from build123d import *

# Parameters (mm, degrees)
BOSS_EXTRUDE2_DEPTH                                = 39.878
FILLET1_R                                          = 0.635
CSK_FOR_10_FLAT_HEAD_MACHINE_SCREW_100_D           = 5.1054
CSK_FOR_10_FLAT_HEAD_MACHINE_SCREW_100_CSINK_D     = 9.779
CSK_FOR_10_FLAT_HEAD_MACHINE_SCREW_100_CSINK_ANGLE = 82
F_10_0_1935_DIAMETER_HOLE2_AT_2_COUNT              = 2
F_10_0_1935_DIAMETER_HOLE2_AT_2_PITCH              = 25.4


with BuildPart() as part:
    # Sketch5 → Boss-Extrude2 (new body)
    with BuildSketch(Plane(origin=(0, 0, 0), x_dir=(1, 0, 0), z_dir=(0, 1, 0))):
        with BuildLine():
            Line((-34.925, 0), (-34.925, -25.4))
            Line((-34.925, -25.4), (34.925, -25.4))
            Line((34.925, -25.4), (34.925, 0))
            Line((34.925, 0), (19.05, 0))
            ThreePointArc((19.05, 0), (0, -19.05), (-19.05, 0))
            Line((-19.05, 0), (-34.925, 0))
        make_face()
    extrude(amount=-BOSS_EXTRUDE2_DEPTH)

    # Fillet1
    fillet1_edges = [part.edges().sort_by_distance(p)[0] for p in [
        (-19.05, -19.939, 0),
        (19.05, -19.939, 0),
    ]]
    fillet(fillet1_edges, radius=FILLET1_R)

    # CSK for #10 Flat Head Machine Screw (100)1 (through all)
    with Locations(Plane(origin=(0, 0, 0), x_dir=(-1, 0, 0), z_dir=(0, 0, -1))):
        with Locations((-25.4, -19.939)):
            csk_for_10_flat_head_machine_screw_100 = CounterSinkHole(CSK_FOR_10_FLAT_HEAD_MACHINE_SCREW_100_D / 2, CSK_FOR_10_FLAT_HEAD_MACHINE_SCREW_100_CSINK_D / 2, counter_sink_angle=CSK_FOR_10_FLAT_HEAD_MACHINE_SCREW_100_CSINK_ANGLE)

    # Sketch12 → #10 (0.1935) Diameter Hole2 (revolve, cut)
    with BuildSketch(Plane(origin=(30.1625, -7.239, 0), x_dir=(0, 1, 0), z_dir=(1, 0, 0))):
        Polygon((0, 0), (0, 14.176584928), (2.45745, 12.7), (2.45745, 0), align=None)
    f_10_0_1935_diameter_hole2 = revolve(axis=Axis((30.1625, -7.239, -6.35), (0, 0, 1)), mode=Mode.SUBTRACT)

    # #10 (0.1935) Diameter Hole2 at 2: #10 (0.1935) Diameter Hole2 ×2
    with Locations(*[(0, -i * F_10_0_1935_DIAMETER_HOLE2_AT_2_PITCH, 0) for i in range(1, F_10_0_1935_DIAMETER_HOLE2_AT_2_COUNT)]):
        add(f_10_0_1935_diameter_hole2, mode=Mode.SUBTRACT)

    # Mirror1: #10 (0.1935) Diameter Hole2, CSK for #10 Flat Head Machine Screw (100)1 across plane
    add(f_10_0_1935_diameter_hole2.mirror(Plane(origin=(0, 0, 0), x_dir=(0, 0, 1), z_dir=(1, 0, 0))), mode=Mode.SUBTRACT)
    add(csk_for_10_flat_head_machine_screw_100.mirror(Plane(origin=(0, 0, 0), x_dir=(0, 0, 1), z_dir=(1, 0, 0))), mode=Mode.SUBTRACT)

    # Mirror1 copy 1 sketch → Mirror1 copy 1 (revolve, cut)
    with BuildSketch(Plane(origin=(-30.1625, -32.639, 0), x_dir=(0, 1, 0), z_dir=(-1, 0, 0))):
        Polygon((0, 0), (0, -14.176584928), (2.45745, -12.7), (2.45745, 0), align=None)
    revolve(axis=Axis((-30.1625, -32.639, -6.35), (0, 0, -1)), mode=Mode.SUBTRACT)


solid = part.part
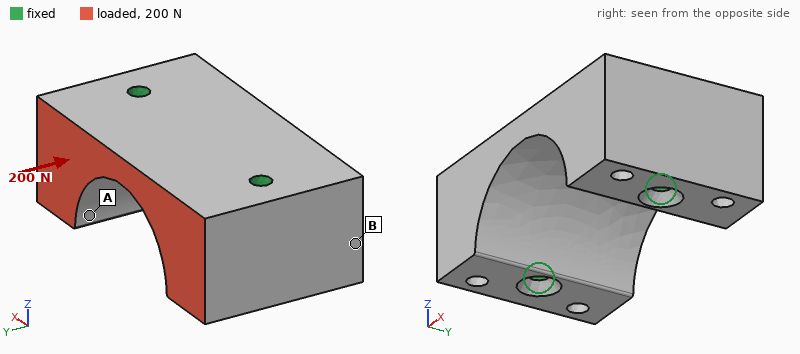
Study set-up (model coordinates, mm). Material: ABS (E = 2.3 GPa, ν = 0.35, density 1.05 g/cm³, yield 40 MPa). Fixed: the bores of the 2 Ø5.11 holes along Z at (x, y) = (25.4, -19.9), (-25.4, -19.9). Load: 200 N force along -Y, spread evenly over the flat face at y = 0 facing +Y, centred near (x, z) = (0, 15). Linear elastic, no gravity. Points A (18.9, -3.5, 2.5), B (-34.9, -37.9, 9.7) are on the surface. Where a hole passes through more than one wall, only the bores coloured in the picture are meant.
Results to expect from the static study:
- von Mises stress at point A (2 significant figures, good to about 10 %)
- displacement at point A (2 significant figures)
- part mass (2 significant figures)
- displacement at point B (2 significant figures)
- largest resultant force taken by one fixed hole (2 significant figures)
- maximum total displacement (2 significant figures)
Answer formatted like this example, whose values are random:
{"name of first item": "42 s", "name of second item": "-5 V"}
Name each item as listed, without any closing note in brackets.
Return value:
{"von Mises stress at point A": "0.15 MPa", "displacement at point A": "1.8 µm", "part mass": "48 g", "displacement at point B": "0.77 µm", "largest resultant force taken by one fixed hole": "100 N", "maximum total displacement": "4.0 µm"}
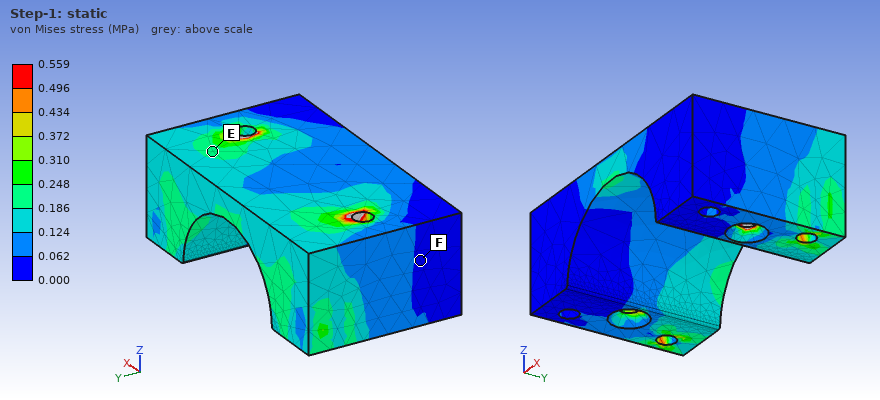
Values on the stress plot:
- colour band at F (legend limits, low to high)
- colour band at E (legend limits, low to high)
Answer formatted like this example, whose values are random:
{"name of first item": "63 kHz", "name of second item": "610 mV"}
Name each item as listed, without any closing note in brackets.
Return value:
{"colour band at F": "0.000 to 0.062 MPa", "colour band at E": "0.186 to 0.248 MPa"}
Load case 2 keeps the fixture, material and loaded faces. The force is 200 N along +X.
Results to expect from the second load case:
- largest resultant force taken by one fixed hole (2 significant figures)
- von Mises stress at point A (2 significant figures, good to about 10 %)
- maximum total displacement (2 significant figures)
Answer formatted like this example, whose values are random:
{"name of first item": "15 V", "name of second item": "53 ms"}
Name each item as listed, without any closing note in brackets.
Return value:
{"largest resultant force taken by one fixed hole": "120 N", "von Mises stress at point A": "0.25 MPa", "maximum total displacement": "14 µm"}
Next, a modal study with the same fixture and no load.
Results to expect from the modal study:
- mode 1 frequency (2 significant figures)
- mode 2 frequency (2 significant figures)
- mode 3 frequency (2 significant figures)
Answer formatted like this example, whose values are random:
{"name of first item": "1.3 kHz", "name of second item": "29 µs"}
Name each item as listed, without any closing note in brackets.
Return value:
{"mode 1 frequency": "5000 Hz", "mode 2 frequency": "6200 Hz", "mode 3 frequency": "6300 Hz"}
